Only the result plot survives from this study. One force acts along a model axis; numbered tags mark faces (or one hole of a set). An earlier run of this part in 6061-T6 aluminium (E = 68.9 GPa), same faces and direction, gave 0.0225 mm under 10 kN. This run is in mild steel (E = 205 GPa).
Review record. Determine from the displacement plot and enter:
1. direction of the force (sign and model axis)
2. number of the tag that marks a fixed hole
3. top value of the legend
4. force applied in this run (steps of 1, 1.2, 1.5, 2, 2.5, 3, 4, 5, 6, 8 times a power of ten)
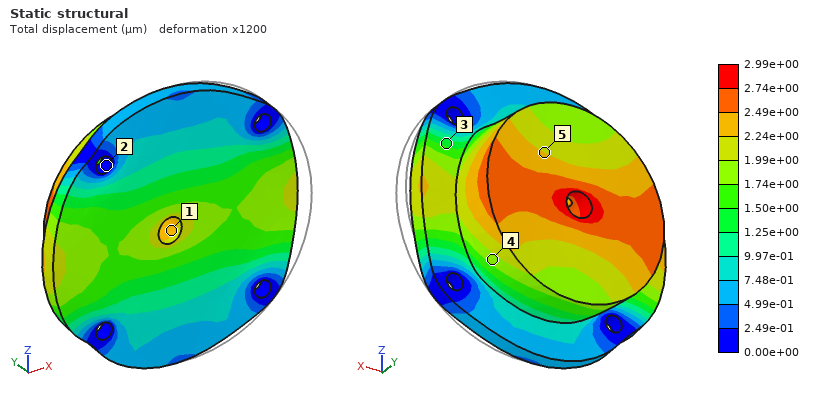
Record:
-X
2
2.99e+00 µm
4 kN
